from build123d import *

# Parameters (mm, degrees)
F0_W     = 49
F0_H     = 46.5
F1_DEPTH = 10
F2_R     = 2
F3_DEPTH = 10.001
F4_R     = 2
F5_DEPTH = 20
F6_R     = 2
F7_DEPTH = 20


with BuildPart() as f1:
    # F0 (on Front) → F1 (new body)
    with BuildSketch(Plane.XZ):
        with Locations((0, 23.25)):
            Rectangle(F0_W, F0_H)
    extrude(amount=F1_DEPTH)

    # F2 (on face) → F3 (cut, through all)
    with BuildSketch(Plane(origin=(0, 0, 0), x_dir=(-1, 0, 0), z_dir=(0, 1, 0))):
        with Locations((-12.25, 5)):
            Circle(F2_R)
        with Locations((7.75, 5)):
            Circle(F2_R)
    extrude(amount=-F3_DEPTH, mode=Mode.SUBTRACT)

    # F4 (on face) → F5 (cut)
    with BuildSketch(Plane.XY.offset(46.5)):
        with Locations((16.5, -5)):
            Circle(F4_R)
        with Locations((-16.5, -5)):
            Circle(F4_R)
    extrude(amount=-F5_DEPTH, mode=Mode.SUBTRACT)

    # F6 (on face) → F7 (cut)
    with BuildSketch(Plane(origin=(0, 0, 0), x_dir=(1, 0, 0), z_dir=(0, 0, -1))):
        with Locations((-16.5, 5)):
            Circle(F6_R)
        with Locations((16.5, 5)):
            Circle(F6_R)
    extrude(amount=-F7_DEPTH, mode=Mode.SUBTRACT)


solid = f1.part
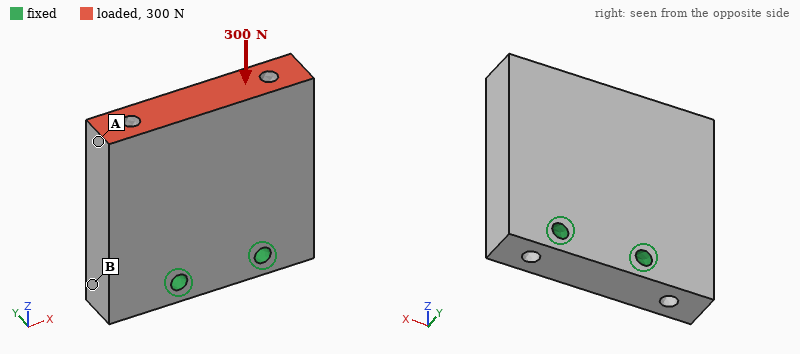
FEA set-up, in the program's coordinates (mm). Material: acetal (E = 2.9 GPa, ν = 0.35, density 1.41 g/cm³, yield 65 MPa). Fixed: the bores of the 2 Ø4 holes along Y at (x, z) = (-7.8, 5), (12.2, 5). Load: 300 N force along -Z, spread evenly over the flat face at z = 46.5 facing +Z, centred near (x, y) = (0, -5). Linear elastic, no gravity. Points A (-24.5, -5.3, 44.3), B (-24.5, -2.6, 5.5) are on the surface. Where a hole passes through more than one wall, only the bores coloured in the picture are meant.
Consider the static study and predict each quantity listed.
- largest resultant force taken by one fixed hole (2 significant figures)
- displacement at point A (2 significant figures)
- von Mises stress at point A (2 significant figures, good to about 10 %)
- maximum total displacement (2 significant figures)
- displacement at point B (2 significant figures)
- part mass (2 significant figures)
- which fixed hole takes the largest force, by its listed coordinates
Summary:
180 N
15 µm
0.65 MPa
16 µm
9.3 µm
30 g
(-7.8, 5)
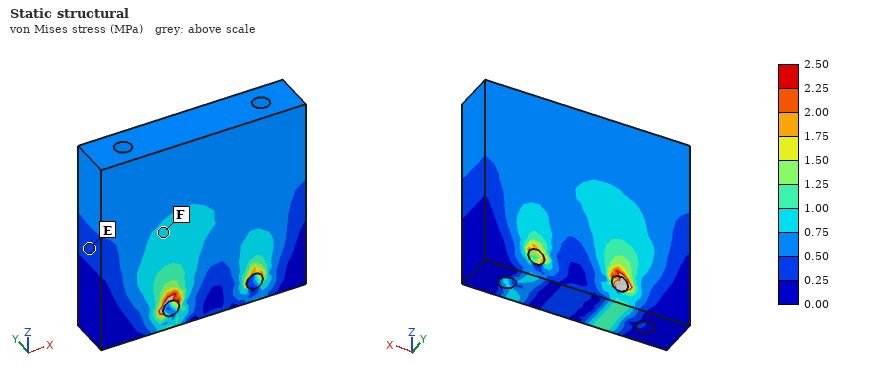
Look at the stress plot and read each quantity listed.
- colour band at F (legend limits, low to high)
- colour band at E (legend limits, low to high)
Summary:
0.75 to 1.00 MPa
0.25 to 0.50 MPa
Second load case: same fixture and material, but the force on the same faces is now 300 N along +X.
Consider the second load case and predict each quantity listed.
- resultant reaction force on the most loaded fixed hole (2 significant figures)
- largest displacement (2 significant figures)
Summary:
560 N
0.14 mm
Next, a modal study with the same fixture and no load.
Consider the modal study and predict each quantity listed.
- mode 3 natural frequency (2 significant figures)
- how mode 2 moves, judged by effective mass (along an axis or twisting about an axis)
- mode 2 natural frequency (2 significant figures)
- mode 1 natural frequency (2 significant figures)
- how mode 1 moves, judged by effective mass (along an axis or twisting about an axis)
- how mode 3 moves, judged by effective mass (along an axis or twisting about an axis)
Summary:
2500 Hz
twisting about Z
2200 Hz
1200 Hz
along Y
along X
